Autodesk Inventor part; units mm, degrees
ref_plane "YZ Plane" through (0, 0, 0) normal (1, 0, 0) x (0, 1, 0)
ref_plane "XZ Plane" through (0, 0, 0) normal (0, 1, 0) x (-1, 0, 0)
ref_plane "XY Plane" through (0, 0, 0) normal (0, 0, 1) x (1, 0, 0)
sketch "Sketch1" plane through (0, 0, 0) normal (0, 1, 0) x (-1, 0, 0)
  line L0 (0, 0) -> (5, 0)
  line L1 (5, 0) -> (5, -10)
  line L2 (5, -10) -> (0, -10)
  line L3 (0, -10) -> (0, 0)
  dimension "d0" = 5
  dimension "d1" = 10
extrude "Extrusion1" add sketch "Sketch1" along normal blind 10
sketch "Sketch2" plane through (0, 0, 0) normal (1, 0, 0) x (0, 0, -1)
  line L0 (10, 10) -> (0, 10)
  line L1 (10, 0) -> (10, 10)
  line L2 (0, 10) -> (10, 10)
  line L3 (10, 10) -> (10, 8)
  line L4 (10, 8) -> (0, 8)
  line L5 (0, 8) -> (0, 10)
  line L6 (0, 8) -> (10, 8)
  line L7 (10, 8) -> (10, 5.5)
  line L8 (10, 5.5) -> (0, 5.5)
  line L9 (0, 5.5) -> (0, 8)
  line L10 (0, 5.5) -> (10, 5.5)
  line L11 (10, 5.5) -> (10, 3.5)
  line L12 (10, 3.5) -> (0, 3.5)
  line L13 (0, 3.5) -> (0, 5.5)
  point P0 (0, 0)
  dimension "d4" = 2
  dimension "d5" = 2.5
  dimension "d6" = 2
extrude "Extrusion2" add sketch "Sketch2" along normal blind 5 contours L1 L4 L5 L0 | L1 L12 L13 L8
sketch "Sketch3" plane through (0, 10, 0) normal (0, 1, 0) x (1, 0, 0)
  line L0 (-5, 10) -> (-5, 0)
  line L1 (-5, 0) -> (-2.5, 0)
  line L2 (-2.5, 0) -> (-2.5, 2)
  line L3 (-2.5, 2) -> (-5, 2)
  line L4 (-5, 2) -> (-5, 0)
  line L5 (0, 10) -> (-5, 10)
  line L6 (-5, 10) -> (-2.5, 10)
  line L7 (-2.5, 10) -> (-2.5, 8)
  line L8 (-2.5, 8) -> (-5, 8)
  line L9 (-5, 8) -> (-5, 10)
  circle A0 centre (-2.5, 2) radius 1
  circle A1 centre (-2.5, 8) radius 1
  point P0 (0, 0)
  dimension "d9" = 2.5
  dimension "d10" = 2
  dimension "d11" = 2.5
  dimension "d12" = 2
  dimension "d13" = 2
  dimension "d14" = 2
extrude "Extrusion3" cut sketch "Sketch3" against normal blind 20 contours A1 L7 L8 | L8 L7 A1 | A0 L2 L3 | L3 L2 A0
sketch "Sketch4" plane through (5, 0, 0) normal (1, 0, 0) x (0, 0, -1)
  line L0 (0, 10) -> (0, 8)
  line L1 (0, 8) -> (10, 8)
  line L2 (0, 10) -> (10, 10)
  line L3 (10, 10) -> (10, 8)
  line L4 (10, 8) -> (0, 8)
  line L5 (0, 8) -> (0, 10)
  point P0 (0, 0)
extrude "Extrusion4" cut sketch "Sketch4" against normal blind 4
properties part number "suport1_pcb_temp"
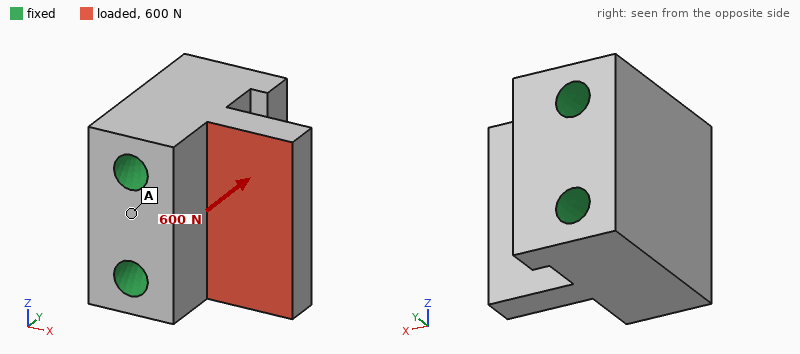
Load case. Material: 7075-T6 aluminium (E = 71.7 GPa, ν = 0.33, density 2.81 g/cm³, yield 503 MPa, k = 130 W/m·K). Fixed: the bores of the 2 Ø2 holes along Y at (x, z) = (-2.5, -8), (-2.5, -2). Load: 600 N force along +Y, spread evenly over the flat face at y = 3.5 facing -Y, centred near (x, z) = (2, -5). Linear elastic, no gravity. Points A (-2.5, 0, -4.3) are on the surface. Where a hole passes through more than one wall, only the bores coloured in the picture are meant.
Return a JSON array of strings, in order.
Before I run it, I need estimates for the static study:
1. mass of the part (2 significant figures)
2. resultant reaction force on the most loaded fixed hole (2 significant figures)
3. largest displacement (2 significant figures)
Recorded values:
["1.6 g", "300 N", "34 µm"]
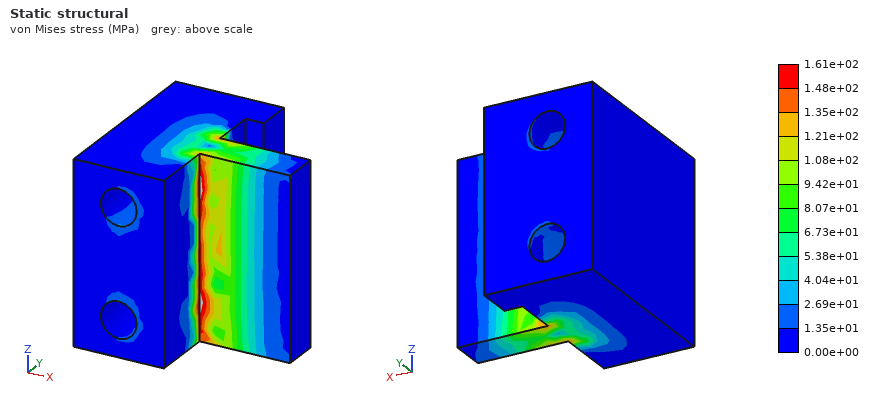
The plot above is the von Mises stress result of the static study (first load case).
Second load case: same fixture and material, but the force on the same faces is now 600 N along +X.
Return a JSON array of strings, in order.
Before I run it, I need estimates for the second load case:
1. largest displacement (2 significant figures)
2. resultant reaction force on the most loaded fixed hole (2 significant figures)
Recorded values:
["15 µm", "310 N"]
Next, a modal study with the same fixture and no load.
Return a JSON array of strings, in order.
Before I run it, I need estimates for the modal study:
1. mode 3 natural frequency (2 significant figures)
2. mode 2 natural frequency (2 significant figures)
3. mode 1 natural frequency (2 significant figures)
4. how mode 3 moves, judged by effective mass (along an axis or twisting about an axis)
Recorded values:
["97 kHz", "72 kHz", "49 kHz", "along Z"]
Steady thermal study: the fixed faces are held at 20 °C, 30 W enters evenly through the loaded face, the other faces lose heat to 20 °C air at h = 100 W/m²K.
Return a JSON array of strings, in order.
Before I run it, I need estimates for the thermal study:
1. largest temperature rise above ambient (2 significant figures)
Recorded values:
["44 K"]
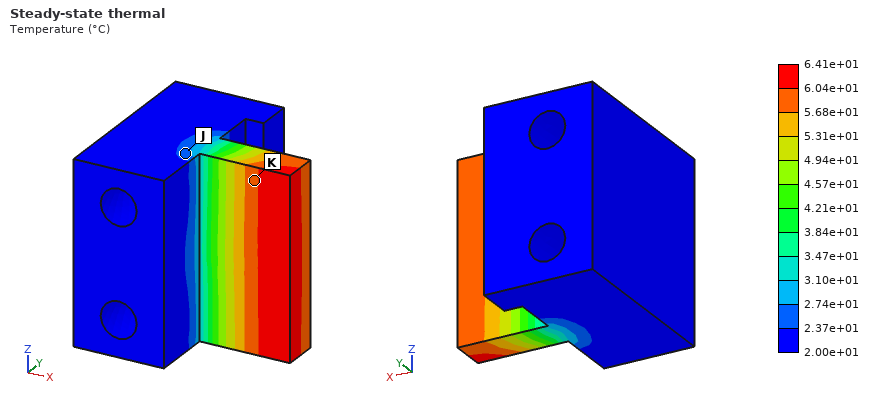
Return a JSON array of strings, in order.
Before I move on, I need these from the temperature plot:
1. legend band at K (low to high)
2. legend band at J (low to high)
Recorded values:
["5.68e+01 to 6.04e+01 °C", "2.37e+01 to 2.74e+01 °C"]
